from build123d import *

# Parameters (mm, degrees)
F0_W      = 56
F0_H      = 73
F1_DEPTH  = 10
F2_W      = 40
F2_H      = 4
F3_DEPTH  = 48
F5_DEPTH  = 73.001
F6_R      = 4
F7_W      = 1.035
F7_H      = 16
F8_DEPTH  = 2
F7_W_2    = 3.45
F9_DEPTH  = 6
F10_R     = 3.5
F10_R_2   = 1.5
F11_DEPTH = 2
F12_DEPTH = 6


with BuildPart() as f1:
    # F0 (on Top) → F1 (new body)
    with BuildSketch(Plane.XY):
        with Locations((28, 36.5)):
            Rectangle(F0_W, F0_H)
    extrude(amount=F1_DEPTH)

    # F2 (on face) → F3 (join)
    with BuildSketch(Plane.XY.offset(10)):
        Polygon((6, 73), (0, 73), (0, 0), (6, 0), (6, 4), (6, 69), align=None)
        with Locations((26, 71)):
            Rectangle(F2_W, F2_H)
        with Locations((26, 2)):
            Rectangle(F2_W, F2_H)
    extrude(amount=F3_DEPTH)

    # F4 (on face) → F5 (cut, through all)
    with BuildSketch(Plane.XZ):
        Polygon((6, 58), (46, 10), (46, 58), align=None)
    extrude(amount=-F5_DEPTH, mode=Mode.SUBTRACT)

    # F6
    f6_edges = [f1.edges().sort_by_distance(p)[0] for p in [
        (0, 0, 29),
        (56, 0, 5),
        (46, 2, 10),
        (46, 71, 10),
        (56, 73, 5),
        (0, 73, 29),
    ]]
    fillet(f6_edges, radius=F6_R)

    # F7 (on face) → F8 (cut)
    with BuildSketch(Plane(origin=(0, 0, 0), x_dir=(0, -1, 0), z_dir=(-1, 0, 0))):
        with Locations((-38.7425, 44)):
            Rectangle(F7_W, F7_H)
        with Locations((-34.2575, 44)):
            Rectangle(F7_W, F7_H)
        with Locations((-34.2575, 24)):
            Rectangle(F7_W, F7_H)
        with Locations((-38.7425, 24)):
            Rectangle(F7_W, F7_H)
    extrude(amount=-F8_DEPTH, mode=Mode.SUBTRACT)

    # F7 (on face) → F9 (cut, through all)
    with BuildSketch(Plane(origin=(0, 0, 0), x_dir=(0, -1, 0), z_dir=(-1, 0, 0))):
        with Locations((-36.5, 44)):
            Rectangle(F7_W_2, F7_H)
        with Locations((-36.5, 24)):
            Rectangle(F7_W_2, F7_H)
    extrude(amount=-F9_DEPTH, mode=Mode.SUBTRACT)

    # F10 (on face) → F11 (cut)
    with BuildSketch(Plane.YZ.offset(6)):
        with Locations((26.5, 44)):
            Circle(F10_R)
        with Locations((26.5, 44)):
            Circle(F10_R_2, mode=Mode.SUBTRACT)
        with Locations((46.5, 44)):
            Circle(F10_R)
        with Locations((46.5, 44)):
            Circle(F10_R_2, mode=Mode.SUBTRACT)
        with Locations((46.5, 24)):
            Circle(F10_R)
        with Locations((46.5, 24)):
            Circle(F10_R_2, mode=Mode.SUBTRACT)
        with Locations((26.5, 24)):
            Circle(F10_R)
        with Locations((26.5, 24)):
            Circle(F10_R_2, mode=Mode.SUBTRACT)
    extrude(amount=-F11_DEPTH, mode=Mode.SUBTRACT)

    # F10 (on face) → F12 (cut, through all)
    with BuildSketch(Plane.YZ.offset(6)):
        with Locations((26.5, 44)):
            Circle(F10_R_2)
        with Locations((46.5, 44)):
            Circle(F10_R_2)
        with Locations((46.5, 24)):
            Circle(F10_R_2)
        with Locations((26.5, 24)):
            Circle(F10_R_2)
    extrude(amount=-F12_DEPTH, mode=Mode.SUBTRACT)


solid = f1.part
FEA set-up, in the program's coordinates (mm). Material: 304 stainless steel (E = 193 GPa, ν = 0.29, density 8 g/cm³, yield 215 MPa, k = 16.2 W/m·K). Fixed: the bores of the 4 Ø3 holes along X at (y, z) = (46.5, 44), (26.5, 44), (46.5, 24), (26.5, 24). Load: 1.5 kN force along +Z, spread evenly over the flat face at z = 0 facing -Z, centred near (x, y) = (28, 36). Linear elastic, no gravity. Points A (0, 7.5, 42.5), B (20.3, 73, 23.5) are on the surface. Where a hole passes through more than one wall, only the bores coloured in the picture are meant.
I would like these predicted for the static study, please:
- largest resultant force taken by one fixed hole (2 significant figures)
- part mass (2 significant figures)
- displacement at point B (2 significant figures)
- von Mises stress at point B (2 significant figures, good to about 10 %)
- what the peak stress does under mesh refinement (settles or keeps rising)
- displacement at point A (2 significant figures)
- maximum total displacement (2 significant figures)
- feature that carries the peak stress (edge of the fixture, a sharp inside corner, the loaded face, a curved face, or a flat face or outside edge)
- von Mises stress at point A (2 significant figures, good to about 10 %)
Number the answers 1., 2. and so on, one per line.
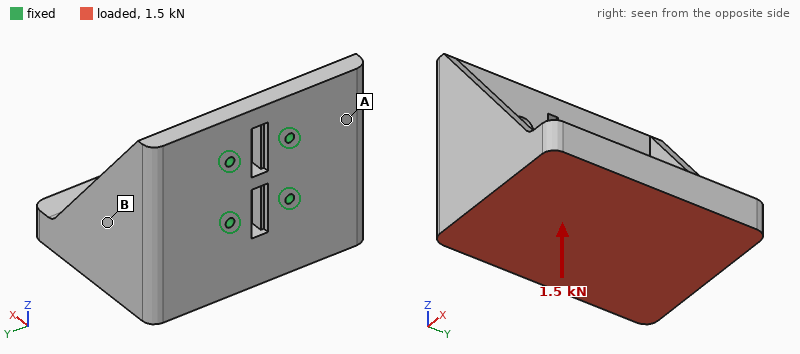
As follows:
1. 990 N
2. 540 g
3. 20 µm
4. 9.5 MPa
5. keeps rising
6. 16 µm
7. 74 µm
8. edge of the fixture
9. 26 MPa
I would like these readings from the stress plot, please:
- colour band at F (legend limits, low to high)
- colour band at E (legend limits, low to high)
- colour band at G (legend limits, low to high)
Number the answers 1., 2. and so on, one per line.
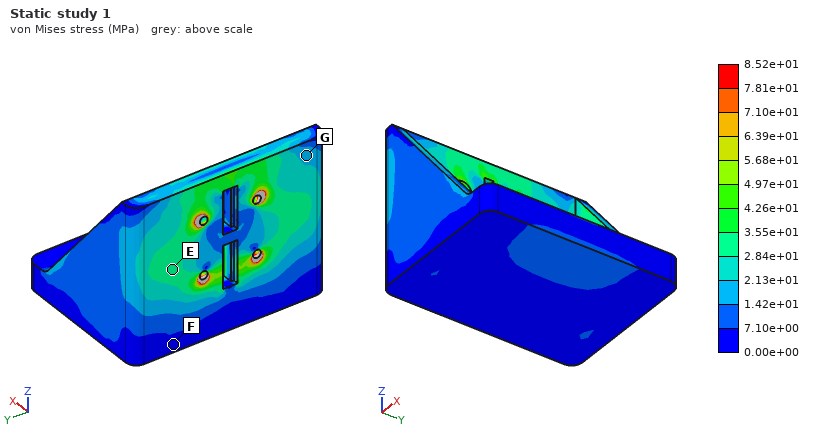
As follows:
1. 0.00e+00 to 7.10e+00 MPa
2. 2.84e+01 to 3.55e+01 MPa
3. 1.42e+01 to 2.13e+01 MPa
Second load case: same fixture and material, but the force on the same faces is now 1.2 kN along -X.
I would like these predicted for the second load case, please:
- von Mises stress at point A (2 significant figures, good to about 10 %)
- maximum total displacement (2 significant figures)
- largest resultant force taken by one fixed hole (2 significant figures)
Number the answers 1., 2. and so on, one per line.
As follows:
1. 18 MPa
2. 50 µm
3. 1.2 kN
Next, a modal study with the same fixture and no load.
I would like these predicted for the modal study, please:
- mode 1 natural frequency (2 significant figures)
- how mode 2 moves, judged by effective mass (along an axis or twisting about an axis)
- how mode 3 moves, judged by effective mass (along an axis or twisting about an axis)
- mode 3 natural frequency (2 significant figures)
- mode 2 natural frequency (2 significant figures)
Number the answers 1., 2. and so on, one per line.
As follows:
1. 1300 Hz
2. along Y
3. along X
4. 3800 Hz
5. 1500 Hz
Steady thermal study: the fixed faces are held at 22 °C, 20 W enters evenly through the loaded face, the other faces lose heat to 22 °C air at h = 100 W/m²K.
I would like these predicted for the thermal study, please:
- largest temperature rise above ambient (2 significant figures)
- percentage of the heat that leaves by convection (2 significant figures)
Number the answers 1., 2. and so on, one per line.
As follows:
1. 25 K
2. 86 %
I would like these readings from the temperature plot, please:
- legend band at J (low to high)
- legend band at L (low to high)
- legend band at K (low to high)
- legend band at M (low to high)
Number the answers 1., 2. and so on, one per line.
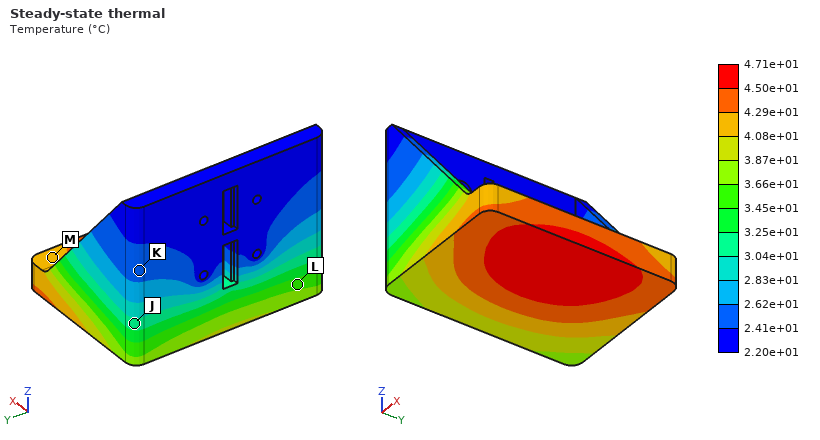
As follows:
1. 3.04e+01 to 3.25e+01 °C
2. 3.45e+01 to 3.66e+01 °C
3. 2.41e+01 to 2.62e+01 °C
4. 4.08e+01 to 4.29e+01 °C
